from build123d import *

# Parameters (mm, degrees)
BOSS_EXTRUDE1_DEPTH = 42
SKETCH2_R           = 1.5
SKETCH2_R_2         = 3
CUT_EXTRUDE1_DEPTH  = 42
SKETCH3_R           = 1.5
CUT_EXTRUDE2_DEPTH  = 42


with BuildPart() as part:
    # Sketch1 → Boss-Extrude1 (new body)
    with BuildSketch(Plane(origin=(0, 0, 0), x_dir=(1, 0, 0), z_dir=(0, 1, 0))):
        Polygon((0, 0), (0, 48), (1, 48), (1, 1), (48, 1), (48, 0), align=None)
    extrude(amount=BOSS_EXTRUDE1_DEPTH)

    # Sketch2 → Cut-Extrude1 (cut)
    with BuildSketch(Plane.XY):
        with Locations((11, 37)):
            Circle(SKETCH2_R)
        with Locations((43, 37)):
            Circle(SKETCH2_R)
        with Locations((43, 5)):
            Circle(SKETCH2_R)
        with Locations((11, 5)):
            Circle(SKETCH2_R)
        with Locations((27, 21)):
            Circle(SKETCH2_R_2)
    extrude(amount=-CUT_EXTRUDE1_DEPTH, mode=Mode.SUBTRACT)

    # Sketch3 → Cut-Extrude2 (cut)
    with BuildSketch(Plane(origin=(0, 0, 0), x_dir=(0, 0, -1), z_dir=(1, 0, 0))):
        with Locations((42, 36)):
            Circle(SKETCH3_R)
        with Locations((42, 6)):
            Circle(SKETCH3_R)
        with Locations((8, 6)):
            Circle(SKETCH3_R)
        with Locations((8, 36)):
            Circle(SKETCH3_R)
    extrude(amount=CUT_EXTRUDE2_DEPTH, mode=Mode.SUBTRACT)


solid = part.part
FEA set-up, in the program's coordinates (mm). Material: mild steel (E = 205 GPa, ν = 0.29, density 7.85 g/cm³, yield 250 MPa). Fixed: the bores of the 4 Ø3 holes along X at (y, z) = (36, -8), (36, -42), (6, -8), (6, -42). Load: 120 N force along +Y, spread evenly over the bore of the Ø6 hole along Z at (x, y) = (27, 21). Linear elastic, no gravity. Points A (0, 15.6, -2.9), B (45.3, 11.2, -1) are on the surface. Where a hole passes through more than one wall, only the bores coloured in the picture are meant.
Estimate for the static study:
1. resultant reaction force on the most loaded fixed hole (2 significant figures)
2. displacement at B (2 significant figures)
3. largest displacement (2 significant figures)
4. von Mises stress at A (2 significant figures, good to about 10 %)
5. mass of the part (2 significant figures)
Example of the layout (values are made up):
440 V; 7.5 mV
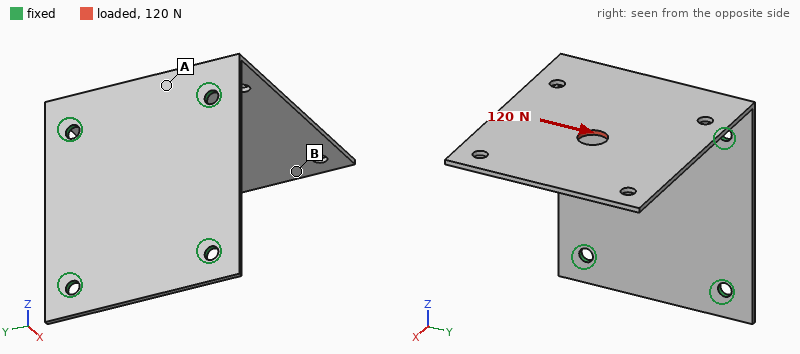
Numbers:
120 N; 0.11 mm; 0.14 mm; 41 MPa; 31 g
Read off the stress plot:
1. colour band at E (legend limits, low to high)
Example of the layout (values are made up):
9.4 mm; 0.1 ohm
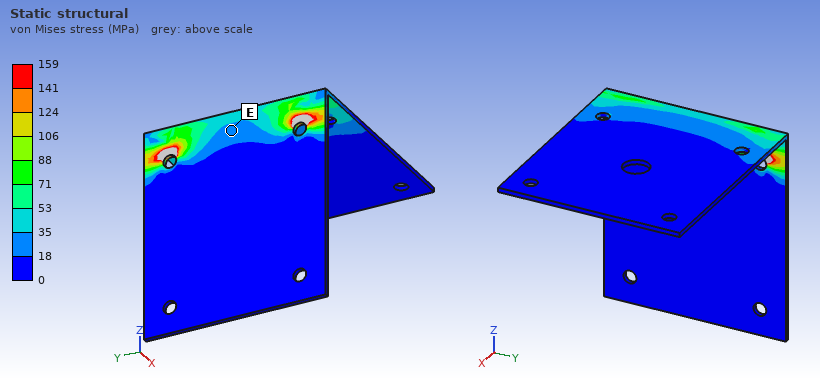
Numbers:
18 to 35 MPa
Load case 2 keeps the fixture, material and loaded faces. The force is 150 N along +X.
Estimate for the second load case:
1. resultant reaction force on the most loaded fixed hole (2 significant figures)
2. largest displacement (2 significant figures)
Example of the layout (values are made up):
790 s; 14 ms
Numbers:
78 N; 0.27 mm
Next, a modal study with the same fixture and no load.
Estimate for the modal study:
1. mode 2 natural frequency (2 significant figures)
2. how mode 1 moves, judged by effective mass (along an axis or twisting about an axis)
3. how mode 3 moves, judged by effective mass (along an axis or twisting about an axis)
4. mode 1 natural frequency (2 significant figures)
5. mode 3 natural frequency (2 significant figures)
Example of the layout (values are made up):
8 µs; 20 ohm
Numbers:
910 Hz; along Z; along Y; 300 Hz; 1700 Hz
